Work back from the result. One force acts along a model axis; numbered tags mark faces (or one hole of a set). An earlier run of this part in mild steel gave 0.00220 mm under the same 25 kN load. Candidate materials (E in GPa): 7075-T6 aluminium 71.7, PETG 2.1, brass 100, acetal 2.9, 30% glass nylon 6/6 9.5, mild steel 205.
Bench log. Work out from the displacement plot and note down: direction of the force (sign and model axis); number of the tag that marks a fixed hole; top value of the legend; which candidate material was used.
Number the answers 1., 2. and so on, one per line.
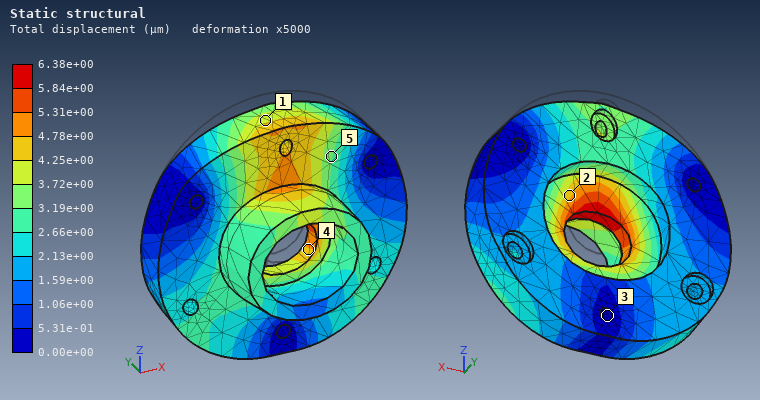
1. -Z
2. 3
3. 6.38e+00 µm
4. 7075-T6 aluminium
